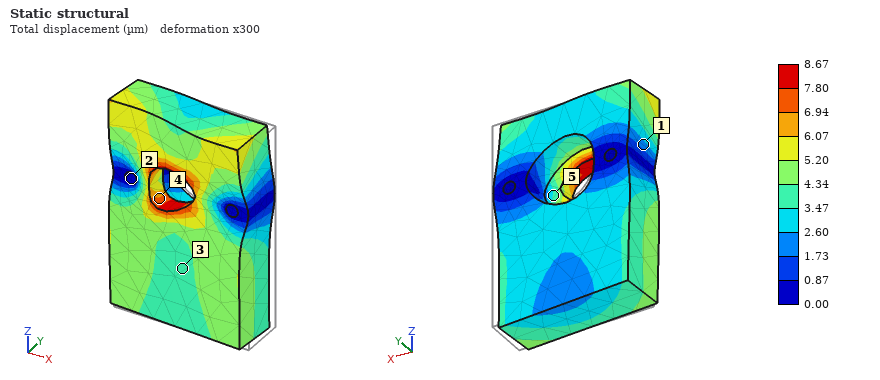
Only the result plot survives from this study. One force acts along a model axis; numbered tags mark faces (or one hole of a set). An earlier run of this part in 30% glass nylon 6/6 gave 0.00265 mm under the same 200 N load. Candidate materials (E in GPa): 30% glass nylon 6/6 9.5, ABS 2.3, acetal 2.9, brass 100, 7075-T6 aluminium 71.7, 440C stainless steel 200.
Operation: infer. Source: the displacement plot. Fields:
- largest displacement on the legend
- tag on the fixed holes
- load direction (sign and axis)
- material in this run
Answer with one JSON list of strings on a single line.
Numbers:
["8.67 µm", "2", "-X", "acetal"]
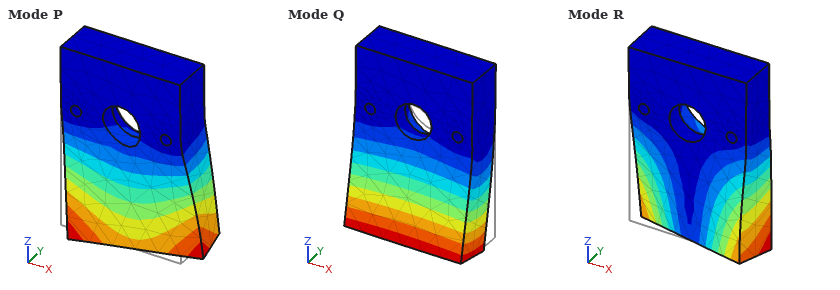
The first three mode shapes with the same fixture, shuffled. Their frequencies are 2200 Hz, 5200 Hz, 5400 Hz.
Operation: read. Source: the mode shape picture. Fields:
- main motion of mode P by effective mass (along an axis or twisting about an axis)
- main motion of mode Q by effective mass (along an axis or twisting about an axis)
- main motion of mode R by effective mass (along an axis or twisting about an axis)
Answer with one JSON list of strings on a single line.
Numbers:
["along X", "along Y", "along X"]
